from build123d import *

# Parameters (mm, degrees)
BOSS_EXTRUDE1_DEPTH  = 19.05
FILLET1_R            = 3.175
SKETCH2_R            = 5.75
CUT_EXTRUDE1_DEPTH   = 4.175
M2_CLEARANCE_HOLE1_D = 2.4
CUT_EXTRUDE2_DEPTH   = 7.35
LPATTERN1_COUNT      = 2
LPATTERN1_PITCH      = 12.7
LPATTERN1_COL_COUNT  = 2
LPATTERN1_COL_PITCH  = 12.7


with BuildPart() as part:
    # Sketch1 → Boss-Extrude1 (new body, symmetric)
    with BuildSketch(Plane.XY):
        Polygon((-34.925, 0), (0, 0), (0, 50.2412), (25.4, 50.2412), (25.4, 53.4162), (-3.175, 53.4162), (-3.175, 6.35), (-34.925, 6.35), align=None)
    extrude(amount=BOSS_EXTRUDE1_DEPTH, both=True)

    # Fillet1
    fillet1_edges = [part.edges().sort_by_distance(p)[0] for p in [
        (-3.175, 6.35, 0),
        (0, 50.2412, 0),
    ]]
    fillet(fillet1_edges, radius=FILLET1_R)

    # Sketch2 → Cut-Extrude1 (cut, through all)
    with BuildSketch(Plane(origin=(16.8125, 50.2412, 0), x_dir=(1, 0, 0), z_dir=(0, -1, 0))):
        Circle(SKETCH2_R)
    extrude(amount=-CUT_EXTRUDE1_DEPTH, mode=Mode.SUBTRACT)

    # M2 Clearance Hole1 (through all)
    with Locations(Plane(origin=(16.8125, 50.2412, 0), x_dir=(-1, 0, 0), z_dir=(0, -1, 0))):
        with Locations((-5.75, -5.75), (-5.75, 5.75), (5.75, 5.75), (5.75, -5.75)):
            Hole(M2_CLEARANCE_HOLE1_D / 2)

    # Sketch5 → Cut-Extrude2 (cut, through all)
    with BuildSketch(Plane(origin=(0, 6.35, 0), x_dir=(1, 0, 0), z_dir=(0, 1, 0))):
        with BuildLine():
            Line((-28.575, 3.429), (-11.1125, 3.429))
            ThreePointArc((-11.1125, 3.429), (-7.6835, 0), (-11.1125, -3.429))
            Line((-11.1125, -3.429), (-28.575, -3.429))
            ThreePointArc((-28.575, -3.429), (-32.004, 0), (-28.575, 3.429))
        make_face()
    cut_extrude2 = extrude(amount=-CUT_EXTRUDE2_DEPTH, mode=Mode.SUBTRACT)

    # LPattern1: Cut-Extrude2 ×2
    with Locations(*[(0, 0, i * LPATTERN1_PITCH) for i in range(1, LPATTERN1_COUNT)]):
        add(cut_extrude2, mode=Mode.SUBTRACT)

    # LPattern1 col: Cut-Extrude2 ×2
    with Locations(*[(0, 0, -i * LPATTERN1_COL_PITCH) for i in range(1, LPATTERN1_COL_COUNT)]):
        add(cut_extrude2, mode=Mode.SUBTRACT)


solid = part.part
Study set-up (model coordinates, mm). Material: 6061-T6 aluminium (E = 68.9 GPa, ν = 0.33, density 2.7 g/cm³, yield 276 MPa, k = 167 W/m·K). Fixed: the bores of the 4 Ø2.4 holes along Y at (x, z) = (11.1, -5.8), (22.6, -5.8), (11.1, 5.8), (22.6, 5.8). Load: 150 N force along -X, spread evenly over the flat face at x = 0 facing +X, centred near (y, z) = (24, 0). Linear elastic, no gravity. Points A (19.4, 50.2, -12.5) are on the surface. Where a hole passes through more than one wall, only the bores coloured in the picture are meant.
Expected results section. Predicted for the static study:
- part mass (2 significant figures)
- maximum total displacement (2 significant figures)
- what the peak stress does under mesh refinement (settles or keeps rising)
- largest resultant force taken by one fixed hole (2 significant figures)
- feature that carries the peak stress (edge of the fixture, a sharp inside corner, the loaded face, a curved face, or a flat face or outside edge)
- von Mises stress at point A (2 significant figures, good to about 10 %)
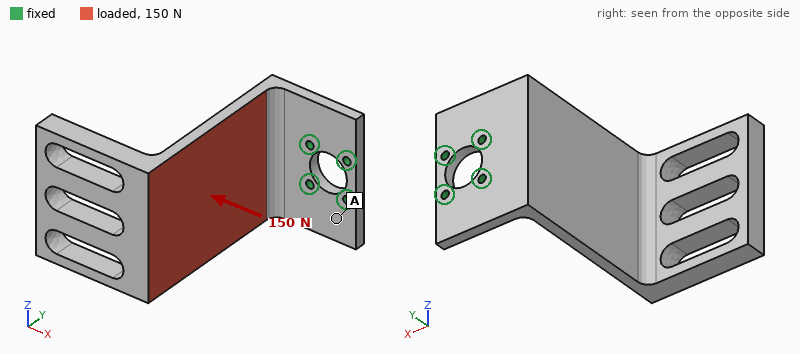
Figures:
38 g
0.90 mm
keeps rising
99 N
edge of the fixture
9.0 MPa
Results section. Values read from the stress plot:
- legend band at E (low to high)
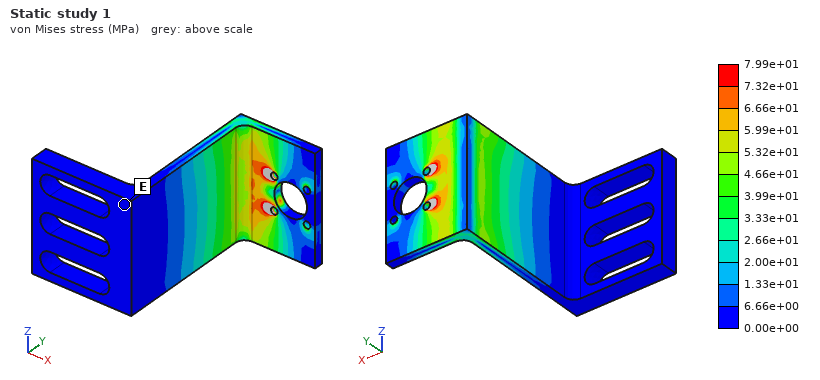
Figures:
0.00e+00 to 6.66e+00 MPa
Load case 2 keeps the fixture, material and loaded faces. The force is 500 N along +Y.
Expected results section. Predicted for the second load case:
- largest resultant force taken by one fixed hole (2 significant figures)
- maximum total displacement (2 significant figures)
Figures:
320 N
0.23 mm
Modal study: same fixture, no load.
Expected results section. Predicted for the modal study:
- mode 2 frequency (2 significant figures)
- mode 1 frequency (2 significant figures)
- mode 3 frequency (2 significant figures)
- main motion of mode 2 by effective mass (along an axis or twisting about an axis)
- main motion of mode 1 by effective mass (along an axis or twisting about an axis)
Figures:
900 Hz
360 Hz
1300 Hz
along Z
along X
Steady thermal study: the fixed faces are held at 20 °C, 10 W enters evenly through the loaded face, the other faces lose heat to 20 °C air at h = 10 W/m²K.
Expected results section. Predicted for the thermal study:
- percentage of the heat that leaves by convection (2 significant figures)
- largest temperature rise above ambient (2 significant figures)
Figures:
9.2 %
18 K
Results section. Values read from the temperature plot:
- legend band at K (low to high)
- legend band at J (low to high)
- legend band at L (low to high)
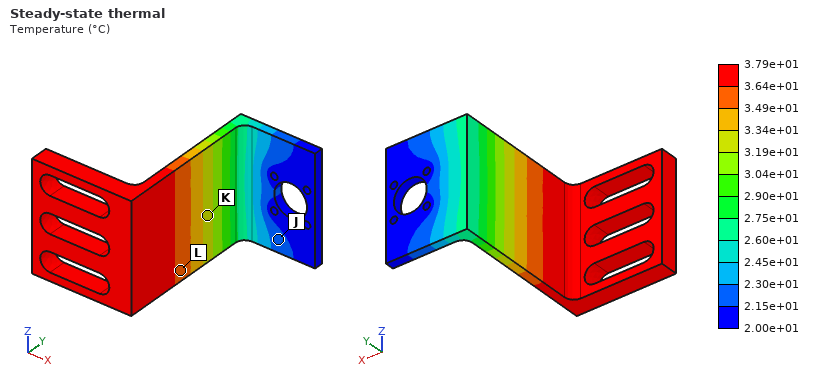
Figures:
3.19e+01 to 3.34e+01 °C
2.15e+01 to 2.30e+01 °C
3.49e+01 to 3.64e+01 °C
